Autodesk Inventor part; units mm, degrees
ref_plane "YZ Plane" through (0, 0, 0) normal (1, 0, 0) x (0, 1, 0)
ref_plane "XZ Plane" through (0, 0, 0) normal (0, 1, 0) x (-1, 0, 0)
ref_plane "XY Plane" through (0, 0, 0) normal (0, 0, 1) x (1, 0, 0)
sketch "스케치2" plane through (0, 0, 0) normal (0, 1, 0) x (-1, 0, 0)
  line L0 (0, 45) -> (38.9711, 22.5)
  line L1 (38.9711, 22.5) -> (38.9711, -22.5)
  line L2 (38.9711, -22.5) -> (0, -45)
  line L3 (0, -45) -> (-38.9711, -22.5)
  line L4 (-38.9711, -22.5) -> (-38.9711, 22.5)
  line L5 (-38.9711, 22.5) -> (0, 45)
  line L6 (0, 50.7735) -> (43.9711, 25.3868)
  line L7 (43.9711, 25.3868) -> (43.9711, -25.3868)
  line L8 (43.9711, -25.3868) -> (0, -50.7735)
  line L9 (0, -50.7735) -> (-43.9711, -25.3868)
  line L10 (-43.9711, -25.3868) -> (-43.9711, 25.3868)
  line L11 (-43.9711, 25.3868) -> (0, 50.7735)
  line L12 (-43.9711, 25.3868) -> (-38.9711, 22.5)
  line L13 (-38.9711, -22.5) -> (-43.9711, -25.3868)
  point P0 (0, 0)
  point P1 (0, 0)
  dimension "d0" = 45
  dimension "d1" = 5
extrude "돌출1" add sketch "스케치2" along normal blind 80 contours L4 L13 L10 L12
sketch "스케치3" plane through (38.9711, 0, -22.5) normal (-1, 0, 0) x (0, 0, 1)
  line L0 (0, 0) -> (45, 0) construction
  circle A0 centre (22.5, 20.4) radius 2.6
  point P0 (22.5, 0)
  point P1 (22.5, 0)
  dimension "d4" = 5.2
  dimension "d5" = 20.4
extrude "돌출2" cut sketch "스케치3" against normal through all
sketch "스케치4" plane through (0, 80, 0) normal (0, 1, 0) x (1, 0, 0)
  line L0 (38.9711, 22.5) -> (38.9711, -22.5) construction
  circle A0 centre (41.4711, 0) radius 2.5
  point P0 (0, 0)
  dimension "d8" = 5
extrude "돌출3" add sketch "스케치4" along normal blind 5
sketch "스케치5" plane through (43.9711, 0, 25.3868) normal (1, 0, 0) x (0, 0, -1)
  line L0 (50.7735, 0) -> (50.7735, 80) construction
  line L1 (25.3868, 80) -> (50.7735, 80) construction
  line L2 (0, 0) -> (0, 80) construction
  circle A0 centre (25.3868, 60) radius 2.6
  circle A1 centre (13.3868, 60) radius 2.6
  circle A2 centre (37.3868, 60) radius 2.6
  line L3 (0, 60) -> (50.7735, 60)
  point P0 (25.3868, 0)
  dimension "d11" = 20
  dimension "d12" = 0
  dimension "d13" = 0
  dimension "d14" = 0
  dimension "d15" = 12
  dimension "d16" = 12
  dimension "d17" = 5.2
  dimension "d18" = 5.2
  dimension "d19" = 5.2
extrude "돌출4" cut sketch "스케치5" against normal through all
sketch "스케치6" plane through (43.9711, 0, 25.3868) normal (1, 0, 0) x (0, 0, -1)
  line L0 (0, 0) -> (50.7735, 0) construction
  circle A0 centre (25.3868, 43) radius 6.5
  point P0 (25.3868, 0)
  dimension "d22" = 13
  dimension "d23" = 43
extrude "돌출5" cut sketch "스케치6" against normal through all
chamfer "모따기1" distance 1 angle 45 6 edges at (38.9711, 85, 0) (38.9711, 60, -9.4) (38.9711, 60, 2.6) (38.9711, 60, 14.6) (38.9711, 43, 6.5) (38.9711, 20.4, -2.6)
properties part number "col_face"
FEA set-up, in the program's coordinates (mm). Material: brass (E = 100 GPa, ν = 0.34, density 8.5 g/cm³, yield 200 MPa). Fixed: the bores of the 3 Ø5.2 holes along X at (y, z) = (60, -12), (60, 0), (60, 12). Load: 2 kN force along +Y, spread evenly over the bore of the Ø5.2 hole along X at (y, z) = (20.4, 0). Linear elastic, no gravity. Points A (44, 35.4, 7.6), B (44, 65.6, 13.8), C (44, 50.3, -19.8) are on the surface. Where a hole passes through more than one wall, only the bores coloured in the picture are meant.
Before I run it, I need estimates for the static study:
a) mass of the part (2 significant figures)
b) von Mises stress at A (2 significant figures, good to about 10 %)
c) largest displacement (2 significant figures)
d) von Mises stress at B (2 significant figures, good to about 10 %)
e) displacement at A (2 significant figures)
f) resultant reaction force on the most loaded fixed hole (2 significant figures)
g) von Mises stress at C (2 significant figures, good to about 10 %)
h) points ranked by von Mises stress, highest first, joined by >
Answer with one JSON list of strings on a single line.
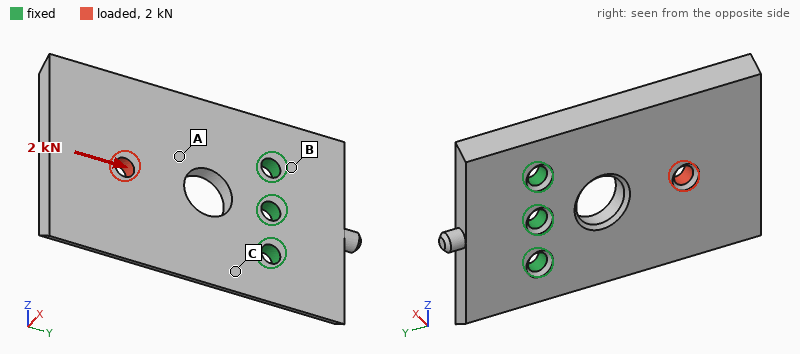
["150 g", "23 MPa", "33 µm", "5.4 MPa", "7.3 µm", "890 N", "13 MPa", "A > C > B"]
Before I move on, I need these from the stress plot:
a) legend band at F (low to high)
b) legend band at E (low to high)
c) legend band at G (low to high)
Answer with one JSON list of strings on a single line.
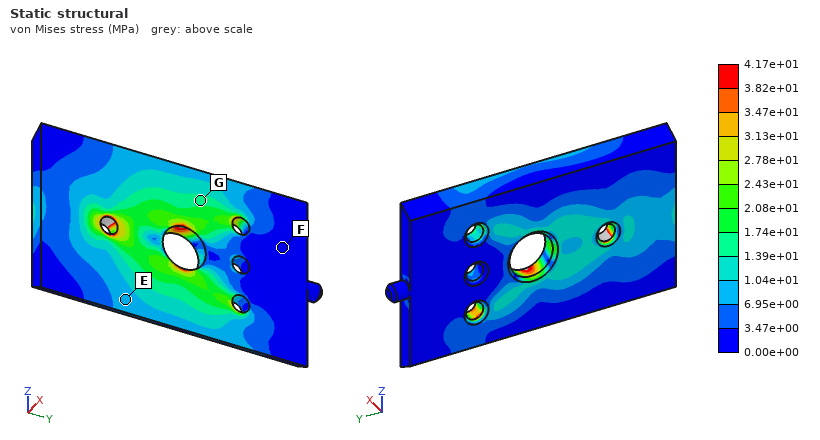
["0.00e+00 to 3.47e+00 MPa", "6.95e+00 to 1.04e+01 MPa", "1.39e+01 to 1.74e+01 MPa"]
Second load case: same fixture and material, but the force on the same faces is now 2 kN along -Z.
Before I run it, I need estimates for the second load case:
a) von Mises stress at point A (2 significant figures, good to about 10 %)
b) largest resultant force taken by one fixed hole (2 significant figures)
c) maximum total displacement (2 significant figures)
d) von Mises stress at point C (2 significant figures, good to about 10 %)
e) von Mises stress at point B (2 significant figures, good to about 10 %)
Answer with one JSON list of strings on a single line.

["25 MPa", "2.8 kN", "49 µm", "26 MPa", "23 MPa"]
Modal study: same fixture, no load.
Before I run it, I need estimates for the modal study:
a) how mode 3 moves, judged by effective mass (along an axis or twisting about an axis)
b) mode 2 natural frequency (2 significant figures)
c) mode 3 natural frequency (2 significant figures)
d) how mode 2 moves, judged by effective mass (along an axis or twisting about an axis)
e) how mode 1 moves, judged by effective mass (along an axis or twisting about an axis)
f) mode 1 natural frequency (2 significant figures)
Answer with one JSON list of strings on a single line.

["along Z", "2000 Hz", "4100 Hz", "twisting about Y", "along X", "720 Hz"]
